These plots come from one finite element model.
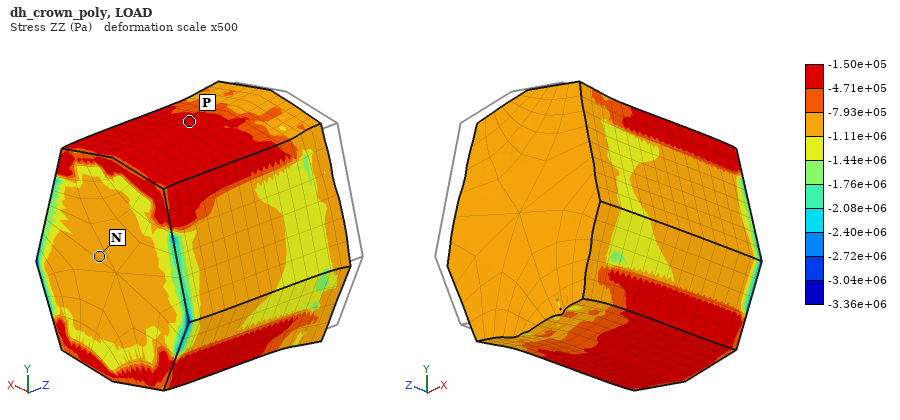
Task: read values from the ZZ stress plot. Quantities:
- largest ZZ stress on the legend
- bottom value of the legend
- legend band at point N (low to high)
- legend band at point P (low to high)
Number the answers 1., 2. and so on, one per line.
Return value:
1. -1.50e+05 Pa
2. -3.36e+06 Pa
3. -1.11e+06 to -7.93e+05 Pa
4. -4.71e+05 to -1.50e+05 Pa
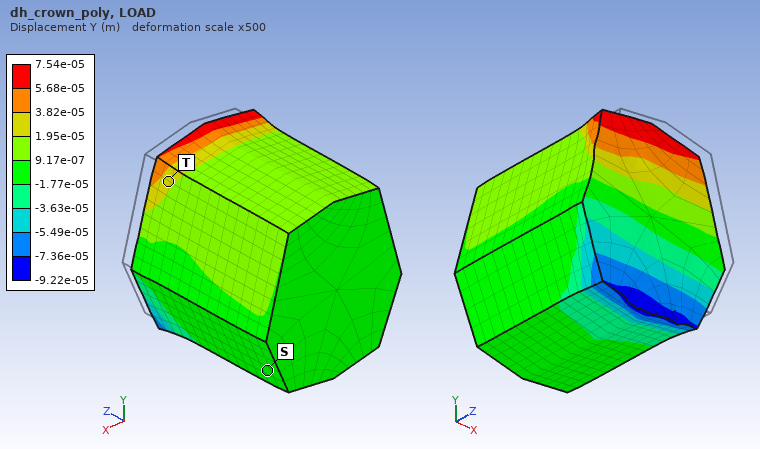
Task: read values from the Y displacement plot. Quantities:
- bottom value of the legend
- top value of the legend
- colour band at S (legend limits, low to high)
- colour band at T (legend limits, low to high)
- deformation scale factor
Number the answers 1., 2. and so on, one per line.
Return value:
1. -9.22e-05 m
2. 7.54e-05 m
3. -1.77e-05 to 9.17e-07 m
4. 1.95e-05 to 3.82e-05 m
5. 500
